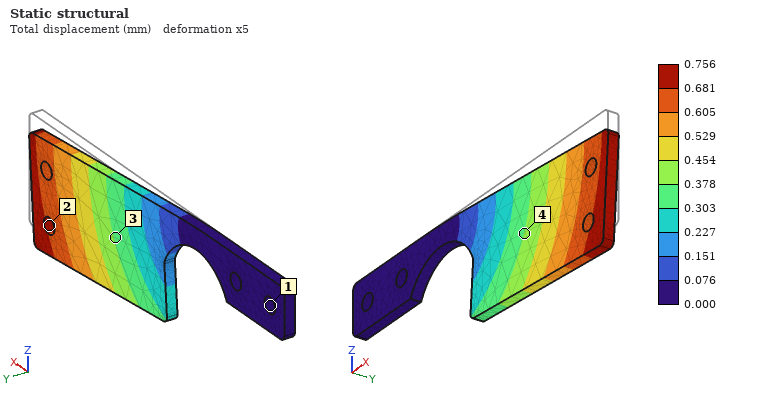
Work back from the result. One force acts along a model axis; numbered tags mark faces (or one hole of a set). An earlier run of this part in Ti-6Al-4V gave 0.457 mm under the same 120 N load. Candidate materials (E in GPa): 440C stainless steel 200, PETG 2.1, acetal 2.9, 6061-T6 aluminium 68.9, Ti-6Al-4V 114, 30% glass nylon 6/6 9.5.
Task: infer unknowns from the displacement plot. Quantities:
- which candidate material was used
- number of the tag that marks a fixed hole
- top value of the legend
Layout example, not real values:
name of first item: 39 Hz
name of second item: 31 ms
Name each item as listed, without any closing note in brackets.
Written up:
which candidate material was used: 6061-T6 aluminium
number of the tag that marks a fixed hole: 1
top value of the legend: 0.756 mm
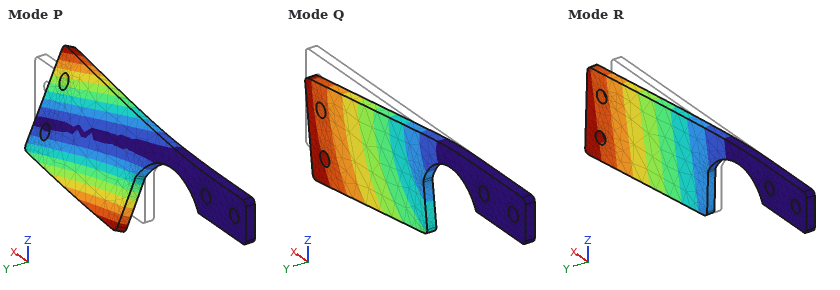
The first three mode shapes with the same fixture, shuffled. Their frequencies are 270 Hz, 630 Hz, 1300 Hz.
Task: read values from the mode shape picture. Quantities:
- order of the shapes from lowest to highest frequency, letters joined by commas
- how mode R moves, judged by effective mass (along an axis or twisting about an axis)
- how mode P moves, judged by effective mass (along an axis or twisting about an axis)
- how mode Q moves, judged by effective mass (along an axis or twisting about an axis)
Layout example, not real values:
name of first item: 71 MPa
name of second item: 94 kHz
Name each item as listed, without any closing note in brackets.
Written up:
order of the shapes from lowest to highest frequency, letters joined by commas: R, Q, P
how mode R moves, judged by effective mass: along Y
how mode P moves, judged by effective mass: twisting about X
how mode Q moves, judged by effective mass: along Z
